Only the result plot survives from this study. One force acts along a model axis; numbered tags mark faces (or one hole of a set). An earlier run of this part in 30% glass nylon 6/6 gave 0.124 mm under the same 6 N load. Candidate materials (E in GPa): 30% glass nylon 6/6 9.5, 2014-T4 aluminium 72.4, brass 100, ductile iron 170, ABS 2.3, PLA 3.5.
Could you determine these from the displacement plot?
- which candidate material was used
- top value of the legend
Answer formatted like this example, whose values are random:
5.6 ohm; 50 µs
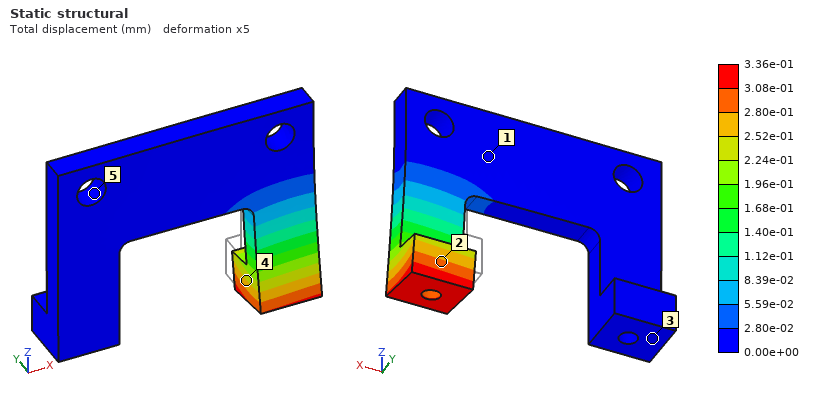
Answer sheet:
PLA; 3.36e-01 mm
